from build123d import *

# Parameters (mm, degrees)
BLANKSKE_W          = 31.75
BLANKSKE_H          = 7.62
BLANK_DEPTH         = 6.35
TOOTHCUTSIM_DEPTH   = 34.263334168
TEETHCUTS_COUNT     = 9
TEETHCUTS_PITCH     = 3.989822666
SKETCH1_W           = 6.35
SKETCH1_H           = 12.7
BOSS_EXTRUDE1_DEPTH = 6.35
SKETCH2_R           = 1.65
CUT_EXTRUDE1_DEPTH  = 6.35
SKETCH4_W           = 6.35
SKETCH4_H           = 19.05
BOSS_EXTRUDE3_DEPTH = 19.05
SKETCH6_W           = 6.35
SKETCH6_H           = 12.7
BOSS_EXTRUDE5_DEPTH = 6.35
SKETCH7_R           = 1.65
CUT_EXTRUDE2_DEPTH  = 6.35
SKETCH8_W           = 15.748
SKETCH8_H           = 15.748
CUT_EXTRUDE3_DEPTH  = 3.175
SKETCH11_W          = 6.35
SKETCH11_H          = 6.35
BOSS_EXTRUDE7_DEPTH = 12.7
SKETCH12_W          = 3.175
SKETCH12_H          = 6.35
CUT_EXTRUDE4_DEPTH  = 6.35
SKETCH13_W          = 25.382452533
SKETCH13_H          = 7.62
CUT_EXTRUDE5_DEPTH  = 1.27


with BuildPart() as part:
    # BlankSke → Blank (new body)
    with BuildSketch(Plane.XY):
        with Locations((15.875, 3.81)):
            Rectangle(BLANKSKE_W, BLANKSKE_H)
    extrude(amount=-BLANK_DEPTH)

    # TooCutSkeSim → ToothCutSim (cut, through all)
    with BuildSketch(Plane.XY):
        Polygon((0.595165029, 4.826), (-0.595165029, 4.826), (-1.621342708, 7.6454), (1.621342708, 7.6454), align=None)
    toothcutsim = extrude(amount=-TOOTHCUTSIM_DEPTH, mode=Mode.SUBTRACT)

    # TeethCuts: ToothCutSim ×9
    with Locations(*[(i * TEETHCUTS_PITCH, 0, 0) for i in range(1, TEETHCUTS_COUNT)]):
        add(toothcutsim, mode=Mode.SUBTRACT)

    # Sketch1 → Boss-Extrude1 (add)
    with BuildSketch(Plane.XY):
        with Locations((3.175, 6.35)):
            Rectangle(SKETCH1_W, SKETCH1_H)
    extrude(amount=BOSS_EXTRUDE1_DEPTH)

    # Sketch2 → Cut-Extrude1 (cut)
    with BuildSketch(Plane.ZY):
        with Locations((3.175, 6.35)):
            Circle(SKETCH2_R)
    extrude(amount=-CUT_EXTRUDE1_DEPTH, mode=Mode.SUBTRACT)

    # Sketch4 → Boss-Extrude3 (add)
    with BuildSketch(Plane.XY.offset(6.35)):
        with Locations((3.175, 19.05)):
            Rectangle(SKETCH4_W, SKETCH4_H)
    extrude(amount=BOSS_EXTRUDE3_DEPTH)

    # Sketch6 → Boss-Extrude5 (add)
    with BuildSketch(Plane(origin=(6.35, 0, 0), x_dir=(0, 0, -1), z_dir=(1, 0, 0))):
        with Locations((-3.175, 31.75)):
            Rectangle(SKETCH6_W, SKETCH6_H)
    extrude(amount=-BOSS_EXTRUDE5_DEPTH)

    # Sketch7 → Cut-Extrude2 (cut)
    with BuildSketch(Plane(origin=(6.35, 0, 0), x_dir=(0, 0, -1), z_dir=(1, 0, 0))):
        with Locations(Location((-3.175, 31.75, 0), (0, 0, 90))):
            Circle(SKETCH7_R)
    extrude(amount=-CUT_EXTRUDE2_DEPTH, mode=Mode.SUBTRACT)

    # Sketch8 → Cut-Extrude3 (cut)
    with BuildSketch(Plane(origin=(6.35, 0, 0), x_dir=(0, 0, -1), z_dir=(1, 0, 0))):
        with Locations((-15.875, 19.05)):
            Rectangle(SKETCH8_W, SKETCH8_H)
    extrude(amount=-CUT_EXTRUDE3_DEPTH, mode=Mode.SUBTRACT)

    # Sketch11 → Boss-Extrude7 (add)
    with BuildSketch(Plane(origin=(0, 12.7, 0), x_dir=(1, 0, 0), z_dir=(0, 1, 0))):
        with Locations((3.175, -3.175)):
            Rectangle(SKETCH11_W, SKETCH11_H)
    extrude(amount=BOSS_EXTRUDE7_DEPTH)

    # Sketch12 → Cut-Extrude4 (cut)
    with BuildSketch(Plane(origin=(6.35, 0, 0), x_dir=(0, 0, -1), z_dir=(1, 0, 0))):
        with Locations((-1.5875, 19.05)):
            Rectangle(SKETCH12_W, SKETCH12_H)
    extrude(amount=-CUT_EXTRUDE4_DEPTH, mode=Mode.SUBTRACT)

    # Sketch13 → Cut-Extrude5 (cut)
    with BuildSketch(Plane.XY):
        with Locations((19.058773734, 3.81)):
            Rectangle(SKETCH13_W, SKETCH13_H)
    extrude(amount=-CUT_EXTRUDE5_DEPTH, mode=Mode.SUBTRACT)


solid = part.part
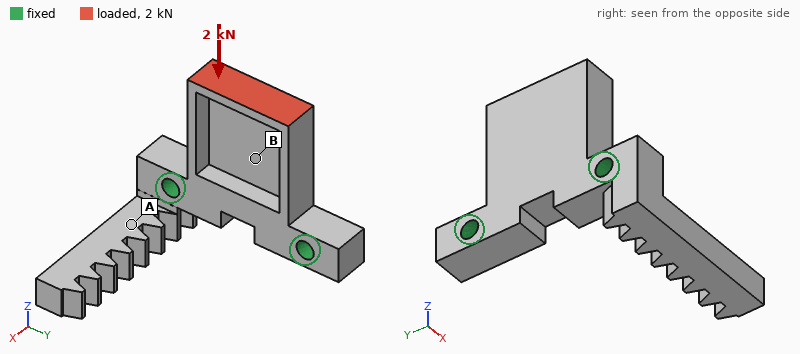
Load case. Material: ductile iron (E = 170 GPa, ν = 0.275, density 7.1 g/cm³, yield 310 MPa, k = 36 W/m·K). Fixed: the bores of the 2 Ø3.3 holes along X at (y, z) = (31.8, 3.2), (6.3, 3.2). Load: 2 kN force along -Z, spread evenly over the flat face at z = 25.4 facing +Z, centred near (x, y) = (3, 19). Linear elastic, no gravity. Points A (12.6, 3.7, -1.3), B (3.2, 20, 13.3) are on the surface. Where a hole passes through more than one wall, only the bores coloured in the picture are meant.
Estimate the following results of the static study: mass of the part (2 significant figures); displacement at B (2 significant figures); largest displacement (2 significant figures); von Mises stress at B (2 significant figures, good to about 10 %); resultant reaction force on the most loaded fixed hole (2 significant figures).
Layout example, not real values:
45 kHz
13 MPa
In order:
27 g
4.8 µm
28 µm
42 MPa
1.1 kN
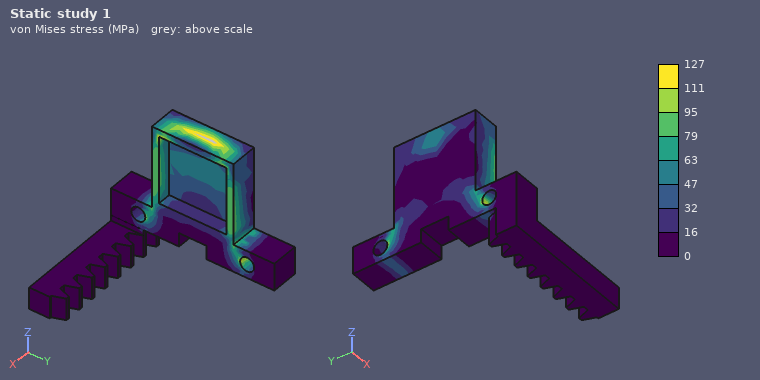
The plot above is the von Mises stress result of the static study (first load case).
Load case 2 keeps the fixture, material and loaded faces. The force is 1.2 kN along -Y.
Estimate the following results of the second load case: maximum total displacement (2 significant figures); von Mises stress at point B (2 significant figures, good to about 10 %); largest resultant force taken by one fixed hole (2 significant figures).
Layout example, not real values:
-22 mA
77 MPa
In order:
42 µm
92 MPa
1.4 kN
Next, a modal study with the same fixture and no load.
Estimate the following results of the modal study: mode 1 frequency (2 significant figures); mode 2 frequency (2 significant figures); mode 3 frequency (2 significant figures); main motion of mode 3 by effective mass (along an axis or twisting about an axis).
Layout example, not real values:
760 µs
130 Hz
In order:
3800 Hz
4000 Hz
6500 Hz
along X
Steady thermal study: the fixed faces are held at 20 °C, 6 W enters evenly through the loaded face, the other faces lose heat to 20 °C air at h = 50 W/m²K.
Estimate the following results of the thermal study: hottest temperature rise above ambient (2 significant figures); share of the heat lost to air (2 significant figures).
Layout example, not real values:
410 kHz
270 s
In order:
50 K
28 %
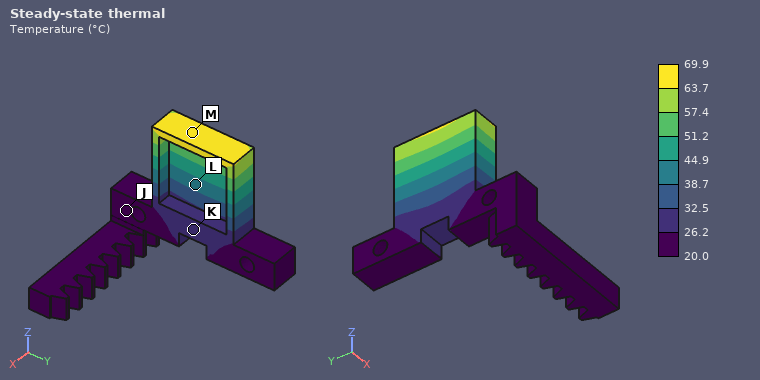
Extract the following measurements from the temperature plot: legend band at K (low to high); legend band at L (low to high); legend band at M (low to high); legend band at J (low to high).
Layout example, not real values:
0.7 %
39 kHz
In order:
26.2 to 32.5 °C
38.7 to 44.9 °C
63.7 to 69.9 °C
20.0 to 26.2 °C
